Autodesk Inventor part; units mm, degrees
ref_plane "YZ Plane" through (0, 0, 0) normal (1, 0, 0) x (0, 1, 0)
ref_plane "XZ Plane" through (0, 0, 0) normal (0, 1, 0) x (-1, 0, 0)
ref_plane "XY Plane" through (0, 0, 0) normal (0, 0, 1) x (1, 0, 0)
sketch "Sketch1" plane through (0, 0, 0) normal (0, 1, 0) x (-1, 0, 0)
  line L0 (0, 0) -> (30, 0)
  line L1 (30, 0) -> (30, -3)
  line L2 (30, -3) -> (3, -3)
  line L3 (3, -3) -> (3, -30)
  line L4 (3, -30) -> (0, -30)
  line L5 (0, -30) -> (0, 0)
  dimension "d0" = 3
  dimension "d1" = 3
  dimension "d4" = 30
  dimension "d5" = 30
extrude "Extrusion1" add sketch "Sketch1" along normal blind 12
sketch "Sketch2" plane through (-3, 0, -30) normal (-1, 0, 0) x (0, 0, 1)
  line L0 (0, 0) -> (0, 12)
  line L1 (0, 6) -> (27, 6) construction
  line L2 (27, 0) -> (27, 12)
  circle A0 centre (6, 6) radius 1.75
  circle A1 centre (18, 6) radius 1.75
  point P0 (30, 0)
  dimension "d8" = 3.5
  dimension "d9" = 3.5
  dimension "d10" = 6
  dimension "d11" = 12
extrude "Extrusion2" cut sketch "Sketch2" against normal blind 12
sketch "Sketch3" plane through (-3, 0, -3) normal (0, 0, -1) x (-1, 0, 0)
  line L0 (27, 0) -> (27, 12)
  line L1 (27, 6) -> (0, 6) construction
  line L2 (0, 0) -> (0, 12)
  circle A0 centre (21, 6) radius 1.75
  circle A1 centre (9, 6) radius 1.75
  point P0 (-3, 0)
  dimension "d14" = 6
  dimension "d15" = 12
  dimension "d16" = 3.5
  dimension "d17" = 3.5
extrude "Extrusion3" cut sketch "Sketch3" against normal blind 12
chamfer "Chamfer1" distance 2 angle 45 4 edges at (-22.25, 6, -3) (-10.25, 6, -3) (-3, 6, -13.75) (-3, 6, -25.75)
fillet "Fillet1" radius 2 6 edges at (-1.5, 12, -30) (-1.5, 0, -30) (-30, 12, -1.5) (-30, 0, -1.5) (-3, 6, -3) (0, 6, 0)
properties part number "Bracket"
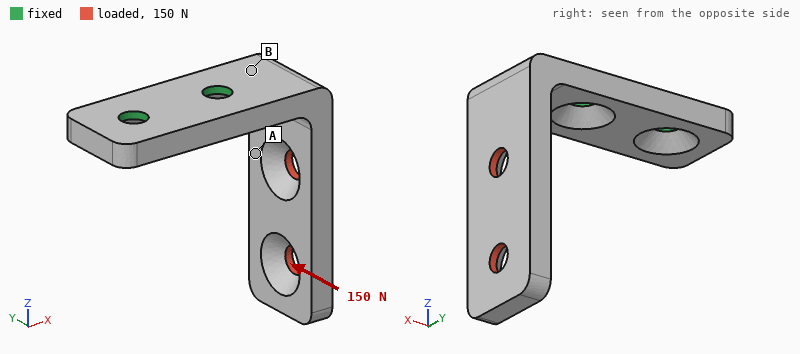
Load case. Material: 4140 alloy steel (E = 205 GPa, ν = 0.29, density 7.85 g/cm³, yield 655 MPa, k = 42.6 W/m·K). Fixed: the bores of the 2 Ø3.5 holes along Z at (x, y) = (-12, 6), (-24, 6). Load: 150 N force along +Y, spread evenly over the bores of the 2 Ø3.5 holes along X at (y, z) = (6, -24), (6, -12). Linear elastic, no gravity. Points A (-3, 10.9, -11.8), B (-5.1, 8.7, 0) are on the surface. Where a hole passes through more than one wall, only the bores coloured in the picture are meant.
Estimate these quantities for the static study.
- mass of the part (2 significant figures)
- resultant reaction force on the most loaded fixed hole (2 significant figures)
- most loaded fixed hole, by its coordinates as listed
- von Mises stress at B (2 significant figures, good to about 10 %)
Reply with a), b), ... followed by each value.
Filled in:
a) 14 g
b) 180 N
c) (-12, 6)
d) 94 MPa
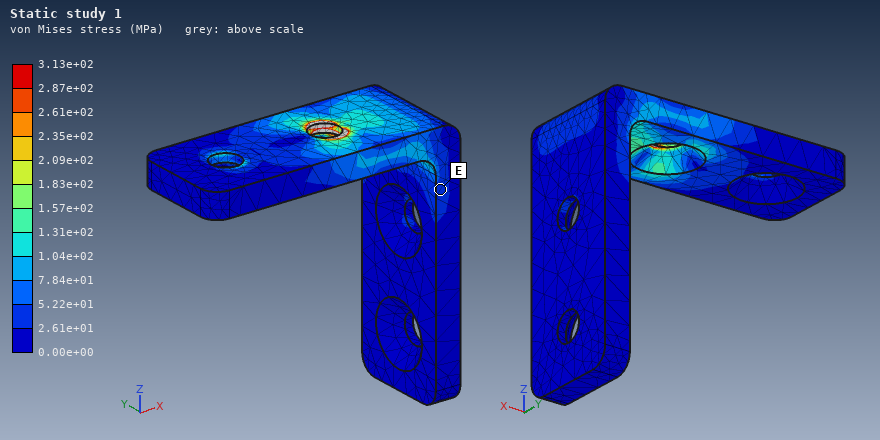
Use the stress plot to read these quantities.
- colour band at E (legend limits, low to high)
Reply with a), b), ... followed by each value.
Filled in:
a) 2.61e+01 to 5.22e+01 MPa
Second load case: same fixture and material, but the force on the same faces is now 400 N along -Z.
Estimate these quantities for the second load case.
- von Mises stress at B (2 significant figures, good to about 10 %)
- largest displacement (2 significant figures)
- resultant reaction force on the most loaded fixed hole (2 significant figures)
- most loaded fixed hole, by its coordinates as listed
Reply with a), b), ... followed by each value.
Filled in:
a) 95 MPa
b) 0.23 mm
c) 830 N
d) (-12, 6)
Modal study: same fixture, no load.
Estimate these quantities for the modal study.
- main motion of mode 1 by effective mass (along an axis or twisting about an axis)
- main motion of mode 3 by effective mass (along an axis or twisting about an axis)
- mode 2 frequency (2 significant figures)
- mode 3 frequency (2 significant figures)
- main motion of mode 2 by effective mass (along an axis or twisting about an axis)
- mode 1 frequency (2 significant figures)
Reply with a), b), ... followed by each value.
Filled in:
a) along X
b) along Z
c) 2600 Hz
d) 7200 Hz
e) along Y
f) 1900 Hz
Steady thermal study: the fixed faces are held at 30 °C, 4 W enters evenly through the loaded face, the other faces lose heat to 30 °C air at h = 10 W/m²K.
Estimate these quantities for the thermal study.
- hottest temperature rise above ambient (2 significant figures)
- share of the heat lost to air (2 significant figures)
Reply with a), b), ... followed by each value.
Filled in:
a) 73 K
b) 13 %
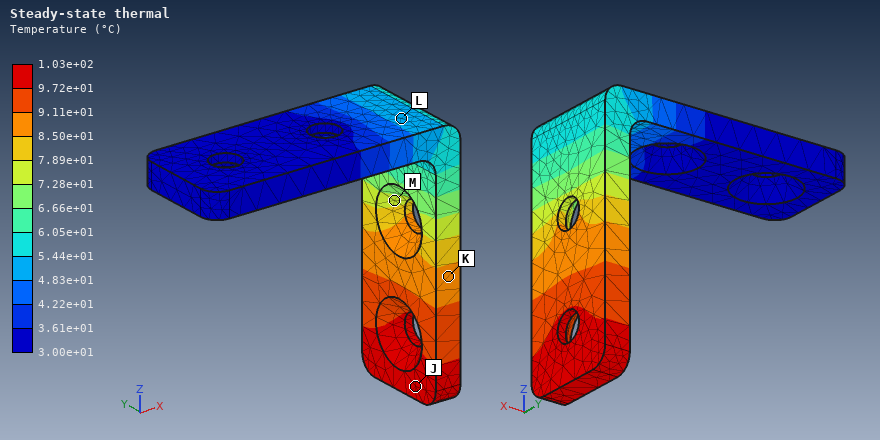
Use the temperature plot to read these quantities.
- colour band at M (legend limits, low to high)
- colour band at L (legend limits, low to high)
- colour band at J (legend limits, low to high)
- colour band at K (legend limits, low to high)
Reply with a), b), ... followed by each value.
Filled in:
a) 7.28e+01 to 7.89e+01 °C
b) 4.83e+01 to 5.44e+01 °C
c) 9.72e+01 to 1.03e+02 °C
d) 8.50e+01 to 9.11e+01 °C
